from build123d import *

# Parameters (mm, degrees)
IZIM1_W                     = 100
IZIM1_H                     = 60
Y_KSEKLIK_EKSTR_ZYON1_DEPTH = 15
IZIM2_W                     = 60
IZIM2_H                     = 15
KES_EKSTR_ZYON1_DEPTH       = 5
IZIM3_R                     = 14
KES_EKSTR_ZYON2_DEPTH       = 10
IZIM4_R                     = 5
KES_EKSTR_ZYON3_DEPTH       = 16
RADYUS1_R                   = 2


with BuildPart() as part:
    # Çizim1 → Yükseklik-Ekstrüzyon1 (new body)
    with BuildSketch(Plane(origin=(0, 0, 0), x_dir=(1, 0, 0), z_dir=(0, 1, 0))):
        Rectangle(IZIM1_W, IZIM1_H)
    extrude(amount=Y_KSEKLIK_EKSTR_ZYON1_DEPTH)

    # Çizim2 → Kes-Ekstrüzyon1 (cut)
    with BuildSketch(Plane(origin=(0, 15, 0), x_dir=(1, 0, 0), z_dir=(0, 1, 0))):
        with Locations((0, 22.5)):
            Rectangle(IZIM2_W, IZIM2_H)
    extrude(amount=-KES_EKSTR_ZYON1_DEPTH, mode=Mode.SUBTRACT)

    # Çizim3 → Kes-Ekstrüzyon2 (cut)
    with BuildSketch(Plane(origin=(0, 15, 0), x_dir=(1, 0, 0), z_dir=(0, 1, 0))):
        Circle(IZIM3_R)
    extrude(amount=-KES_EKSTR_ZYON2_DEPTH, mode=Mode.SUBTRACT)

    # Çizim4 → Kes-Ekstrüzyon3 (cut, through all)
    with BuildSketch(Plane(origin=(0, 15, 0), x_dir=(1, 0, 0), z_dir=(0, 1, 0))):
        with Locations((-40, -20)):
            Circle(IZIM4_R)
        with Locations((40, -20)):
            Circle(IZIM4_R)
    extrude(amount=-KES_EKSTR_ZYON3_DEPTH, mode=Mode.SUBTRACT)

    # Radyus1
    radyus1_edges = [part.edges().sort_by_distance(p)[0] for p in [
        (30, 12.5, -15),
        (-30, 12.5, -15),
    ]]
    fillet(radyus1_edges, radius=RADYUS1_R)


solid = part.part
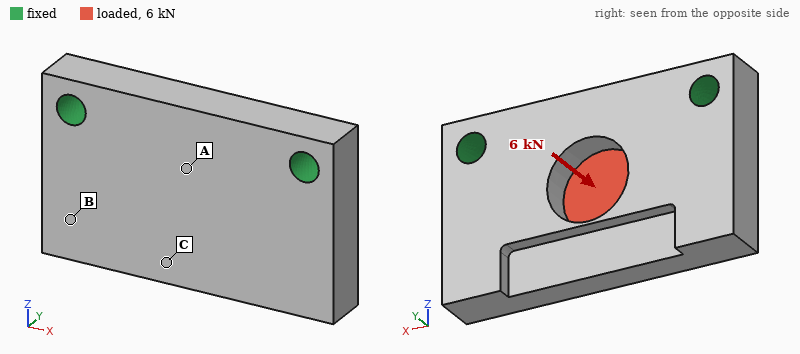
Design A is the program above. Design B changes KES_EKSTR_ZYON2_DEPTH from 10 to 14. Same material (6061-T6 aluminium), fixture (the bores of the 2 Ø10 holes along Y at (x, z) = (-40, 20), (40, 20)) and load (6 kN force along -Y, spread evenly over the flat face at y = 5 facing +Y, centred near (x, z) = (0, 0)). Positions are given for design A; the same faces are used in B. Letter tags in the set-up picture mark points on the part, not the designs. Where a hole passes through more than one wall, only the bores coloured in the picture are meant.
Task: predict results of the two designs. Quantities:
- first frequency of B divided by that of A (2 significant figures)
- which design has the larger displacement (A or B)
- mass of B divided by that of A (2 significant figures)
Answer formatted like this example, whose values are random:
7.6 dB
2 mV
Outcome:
1.0
B
0.97
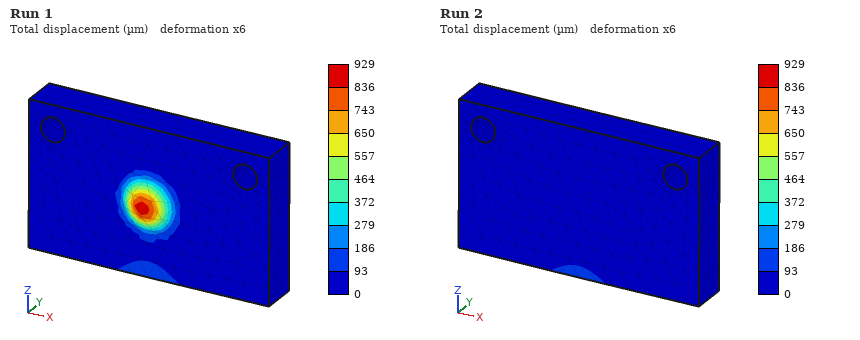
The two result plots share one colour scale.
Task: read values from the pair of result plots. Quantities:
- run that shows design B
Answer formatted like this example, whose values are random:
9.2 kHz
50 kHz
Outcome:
Run 1
